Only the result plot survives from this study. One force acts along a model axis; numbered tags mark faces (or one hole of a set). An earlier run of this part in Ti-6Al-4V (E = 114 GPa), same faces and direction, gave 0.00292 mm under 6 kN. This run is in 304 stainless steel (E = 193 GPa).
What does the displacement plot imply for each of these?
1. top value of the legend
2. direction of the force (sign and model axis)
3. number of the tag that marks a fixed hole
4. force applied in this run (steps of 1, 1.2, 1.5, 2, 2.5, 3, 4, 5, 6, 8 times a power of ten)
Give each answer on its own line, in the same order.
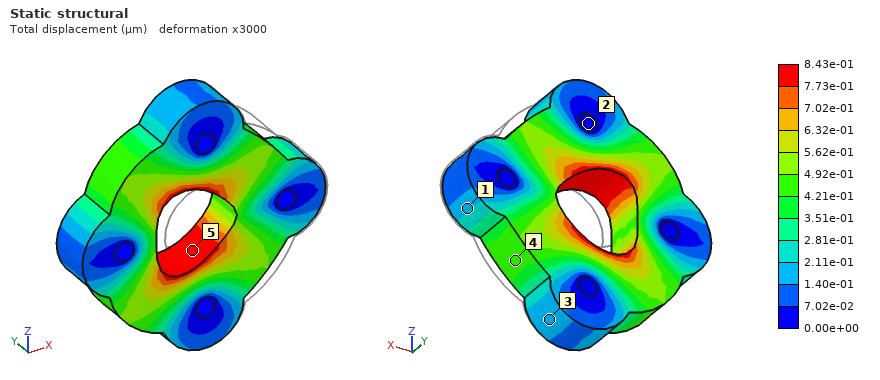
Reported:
8.43e-01 µm
-X
2
3 kN
